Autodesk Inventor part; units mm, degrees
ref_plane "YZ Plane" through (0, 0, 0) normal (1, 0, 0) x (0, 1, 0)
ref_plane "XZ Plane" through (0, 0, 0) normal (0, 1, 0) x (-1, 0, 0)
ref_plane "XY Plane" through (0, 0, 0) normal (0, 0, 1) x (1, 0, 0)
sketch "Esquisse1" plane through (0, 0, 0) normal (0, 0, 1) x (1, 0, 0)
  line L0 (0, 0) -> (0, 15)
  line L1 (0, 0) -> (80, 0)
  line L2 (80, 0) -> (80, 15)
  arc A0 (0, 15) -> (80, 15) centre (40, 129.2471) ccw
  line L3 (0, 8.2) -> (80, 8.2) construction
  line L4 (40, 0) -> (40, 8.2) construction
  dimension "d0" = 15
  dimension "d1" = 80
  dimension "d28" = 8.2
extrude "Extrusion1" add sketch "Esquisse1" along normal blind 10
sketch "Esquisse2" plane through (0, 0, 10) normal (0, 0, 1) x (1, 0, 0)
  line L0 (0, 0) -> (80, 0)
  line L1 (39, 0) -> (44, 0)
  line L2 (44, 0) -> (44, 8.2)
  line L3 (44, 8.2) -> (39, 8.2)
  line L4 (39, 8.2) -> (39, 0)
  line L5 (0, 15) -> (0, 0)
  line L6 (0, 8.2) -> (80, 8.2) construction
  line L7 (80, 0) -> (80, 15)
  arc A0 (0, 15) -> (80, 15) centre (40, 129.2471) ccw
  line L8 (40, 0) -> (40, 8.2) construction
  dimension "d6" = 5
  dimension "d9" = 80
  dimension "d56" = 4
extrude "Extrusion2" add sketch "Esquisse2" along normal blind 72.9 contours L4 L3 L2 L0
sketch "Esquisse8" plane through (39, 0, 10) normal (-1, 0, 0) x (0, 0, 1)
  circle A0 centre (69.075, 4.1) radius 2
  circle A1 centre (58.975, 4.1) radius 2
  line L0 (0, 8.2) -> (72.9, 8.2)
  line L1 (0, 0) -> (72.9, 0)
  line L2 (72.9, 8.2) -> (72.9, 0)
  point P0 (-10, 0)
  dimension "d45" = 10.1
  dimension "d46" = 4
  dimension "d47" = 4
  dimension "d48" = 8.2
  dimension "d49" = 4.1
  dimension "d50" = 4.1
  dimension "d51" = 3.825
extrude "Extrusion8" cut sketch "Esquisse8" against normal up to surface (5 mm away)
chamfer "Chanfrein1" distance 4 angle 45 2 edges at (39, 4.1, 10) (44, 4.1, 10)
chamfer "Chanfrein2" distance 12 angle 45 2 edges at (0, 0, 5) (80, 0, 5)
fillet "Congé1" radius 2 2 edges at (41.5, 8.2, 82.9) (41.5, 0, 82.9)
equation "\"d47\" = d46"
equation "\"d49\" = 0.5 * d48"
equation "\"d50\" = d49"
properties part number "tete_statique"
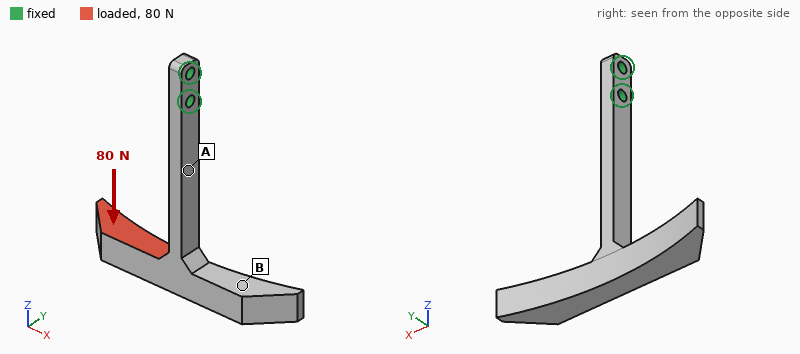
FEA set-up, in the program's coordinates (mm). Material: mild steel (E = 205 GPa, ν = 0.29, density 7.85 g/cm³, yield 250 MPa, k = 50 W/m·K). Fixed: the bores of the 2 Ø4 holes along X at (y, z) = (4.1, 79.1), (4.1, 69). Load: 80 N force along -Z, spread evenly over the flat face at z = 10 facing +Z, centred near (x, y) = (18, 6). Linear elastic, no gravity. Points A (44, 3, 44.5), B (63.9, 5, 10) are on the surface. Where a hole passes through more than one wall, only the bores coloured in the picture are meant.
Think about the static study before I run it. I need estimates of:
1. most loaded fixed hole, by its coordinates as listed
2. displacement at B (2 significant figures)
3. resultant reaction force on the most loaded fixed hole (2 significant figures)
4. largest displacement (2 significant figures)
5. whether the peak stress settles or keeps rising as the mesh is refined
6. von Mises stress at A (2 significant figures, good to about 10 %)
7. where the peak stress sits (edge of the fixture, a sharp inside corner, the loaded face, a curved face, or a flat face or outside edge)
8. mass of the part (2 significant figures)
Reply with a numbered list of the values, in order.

1. (4.1, 69)
2. 0.22 mm
3. 78 N
4. 0.34 mm
5. keeps rising
6. 53 MPa
7. edge of the fixture
8. 78 g
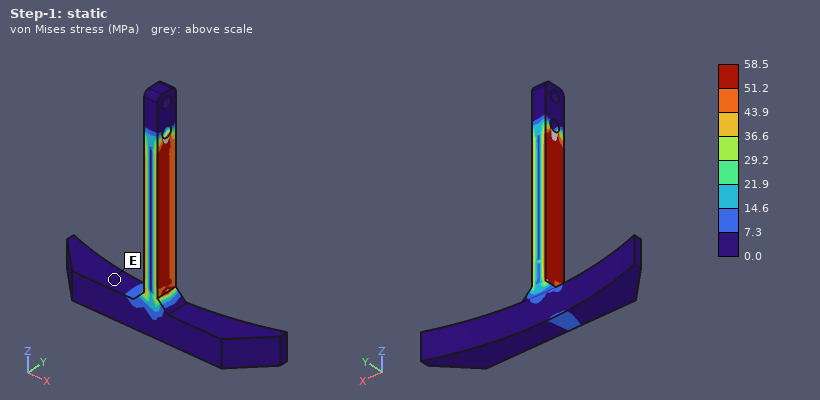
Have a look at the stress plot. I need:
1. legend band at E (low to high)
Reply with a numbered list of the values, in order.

1. 0.0 to 7.3 MPa
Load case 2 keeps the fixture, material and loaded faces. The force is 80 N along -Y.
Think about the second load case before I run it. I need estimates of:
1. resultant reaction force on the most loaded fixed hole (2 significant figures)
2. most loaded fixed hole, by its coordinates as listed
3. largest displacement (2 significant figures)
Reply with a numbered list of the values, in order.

1. 170 N
2. (4.1, 69)
3. 0.41 mm
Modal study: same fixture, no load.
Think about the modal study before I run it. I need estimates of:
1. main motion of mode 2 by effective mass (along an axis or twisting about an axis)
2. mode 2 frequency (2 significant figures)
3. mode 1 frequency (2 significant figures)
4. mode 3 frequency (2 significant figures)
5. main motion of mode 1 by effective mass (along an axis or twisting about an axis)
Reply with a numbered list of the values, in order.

1. along Y
2. 470 Hz
3. 270 Hz
4. 540 Hz
5. along X
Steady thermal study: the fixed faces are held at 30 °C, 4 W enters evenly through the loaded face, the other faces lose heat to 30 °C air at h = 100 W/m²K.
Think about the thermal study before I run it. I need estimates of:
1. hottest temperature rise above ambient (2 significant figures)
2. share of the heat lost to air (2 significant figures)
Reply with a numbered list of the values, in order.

1. 20 K
2. 95 %
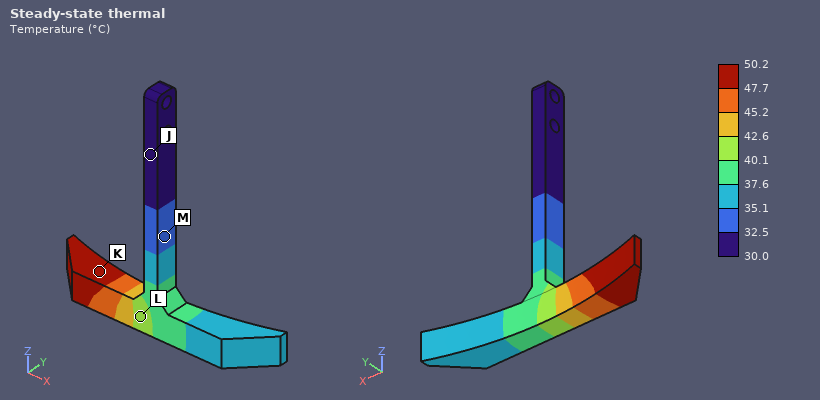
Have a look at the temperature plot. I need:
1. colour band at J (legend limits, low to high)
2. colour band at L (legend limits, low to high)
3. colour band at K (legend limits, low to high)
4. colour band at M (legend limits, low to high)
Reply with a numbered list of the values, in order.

1. 30.0 to 32.5 °C
2. 40.1 to 42.6 °C
3. 47.7 to 50.2 °C
4. 32.5 to 35.1 °C
